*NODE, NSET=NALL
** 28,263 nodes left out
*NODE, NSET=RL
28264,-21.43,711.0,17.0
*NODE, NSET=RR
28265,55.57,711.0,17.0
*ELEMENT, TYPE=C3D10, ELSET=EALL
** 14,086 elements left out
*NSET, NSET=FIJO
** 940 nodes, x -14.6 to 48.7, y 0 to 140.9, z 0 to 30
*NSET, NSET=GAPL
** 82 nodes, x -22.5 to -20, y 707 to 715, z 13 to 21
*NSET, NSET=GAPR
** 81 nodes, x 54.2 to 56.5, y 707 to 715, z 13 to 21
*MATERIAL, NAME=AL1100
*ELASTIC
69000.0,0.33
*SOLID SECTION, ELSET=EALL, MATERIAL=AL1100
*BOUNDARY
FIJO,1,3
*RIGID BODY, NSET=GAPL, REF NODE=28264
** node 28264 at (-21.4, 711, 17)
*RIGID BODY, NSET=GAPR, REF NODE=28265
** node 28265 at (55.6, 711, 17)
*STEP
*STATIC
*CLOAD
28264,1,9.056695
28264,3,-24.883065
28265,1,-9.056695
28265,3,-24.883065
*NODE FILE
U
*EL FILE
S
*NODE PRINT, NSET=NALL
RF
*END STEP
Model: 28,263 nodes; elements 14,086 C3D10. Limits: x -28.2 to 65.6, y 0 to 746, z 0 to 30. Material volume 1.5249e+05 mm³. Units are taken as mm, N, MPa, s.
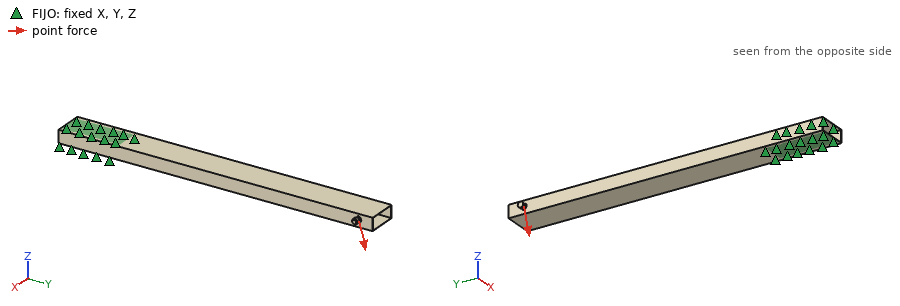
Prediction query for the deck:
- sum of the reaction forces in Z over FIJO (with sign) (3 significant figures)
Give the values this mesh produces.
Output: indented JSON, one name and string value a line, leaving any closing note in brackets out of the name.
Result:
{
  "sum of the reaction forces in Z over FIJO (with sign)": "49.8 N"
}
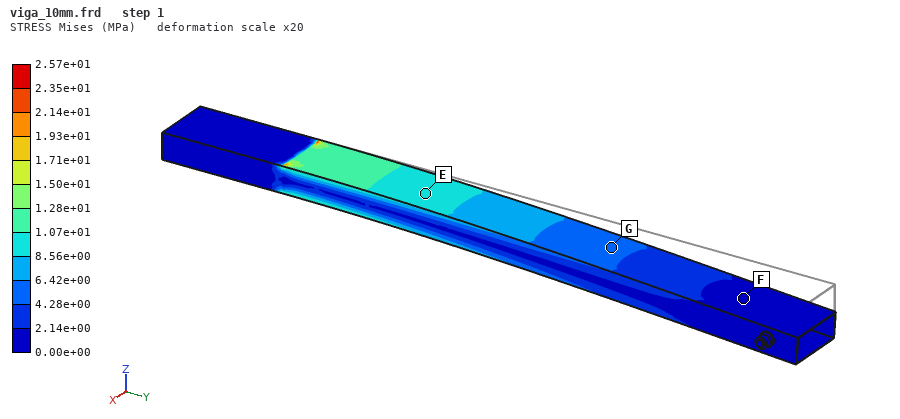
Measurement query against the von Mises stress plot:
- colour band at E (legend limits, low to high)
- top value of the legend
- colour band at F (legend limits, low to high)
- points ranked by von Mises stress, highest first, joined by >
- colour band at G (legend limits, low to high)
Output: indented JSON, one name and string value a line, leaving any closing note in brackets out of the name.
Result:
{
  "colour band at E": "8.56e+00 to 1.07e+01 MPa",
  "top value of the legend": "2.57e+01 MPa",
  "colour band at F": "0.00e+00 to 2.14e+00 MPa",
  "points ranked by von Mises stress, highest first, joined by >": "E > G > F",
  "colour band at G": "4.28e+00 to 6.42e+00 MPa"
}
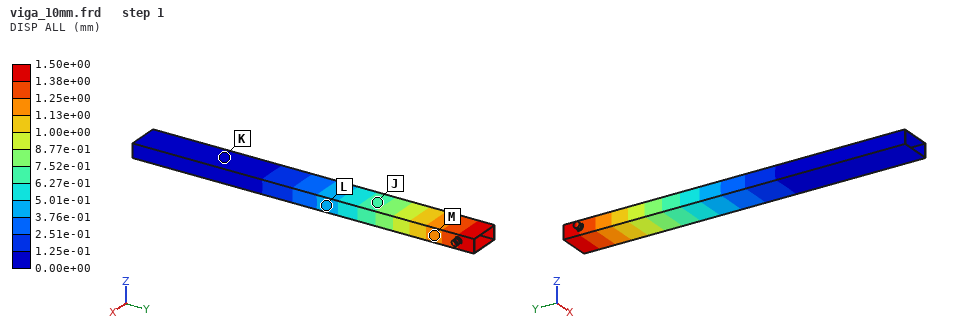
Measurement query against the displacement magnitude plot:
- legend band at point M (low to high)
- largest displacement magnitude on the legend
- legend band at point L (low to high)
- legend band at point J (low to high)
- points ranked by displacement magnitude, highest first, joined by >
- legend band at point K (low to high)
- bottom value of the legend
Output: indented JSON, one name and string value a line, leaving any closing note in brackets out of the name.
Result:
{
  "legend band at point M": "1.13e+00 to 1.25e+00 mm",
  "largest displacement magnitude on the legend": "1.50e+00 mm",
  "legend band at point L": "3.76e-01 to 5.01e-01 mm",
  "legend band at point J": "6.27e-01 to 7.52e-01 mm",
  "points ranked by displacement magnitude, highest first, joined by >": "M > J > L > K",
  "legend band at point K": "0.00e+00 to 1.25e-01 mm",
  "bottom value of the legend": "0.00e+00 mm"
}
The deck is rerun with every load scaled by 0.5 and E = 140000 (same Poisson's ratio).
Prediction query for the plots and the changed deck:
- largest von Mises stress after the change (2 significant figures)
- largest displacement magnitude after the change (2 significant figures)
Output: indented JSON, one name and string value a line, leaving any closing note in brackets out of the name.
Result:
{
  "largest von Mises stress after the change": "13 MPa",
  "largest displacement magnitude after the change": "0.37 mm"
}
